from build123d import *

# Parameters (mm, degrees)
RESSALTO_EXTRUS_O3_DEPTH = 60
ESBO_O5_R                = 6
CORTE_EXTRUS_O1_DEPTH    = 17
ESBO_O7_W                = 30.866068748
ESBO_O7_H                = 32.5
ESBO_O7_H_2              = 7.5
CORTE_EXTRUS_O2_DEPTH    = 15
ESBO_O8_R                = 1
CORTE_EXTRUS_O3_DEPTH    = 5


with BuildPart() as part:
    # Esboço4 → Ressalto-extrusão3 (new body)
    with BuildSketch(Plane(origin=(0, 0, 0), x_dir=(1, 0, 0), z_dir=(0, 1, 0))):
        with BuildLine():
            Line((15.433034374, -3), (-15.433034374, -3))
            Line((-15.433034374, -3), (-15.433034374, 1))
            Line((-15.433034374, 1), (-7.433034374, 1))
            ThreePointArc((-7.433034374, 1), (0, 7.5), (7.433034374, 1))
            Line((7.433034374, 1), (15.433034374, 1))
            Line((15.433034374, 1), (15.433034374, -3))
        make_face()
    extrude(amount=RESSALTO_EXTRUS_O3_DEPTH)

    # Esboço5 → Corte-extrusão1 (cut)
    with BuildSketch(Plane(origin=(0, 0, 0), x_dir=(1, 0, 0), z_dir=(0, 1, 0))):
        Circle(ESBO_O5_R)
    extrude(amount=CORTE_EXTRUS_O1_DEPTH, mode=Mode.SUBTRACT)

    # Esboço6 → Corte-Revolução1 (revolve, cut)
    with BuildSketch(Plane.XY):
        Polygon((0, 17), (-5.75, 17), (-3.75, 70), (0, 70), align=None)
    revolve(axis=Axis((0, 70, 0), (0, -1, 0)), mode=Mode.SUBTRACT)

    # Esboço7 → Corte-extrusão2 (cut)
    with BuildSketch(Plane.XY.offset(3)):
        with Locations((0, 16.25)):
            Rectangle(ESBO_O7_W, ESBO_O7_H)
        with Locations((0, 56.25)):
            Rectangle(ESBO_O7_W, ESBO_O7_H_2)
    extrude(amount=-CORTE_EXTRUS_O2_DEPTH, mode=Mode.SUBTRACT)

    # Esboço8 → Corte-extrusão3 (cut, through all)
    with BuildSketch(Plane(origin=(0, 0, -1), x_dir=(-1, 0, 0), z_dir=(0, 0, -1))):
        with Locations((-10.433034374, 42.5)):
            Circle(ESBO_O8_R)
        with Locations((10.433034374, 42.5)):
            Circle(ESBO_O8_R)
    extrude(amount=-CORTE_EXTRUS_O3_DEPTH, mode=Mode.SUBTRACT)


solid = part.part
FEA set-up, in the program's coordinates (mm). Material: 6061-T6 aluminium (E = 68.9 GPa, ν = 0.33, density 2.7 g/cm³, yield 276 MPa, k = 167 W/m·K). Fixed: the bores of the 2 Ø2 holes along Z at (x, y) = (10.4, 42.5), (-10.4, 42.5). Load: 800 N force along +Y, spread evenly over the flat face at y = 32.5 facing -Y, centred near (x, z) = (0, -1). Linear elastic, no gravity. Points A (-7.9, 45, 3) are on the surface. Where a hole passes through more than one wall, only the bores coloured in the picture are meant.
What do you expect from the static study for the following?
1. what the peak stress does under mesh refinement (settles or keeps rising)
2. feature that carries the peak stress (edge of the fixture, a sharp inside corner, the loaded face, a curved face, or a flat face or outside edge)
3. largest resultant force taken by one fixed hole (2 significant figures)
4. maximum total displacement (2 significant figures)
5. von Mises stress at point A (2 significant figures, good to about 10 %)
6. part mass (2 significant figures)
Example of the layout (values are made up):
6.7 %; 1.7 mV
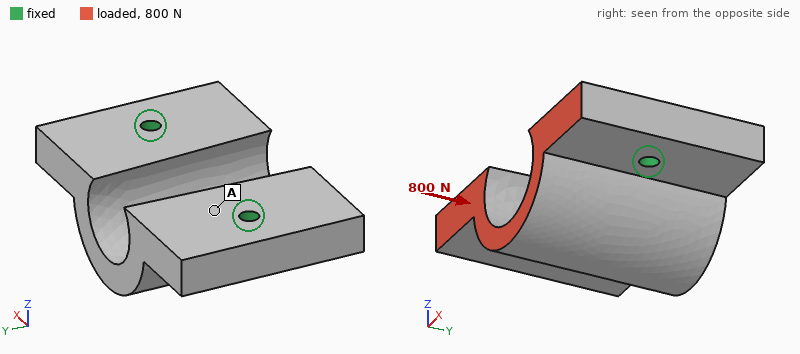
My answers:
keeps rising; edge of the fixture; 400 N; 13 µm; 6.3 MPa; 7.2 g
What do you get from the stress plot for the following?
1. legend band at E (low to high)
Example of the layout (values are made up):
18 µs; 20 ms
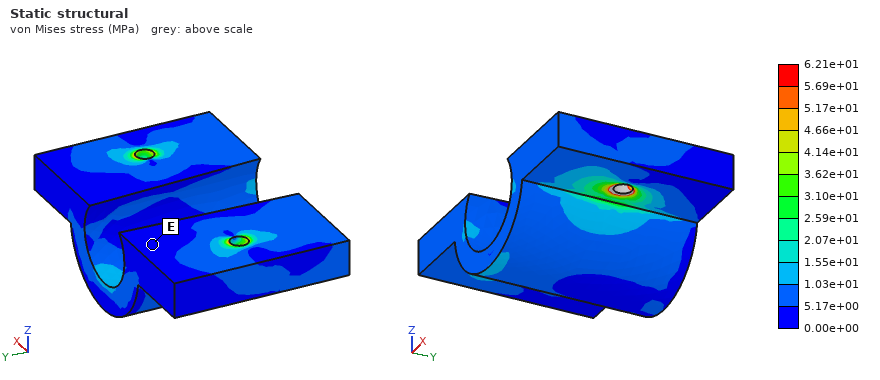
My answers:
0.00e+00 to 5.17e+00 MPa
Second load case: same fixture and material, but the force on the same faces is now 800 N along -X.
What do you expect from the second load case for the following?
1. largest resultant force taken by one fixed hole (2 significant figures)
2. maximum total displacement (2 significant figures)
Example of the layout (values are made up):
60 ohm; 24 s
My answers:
490 N; 19 µm
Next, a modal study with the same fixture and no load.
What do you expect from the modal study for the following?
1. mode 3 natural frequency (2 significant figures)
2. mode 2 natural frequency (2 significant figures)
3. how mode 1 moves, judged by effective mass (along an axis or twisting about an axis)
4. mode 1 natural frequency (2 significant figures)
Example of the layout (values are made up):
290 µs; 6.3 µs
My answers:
24 kHz; 22 kHz; along Y; 14 kHz
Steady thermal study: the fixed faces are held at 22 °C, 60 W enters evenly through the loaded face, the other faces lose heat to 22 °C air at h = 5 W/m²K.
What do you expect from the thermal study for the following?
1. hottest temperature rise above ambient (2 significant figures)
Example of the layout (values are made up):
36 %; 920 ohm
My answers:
40 K
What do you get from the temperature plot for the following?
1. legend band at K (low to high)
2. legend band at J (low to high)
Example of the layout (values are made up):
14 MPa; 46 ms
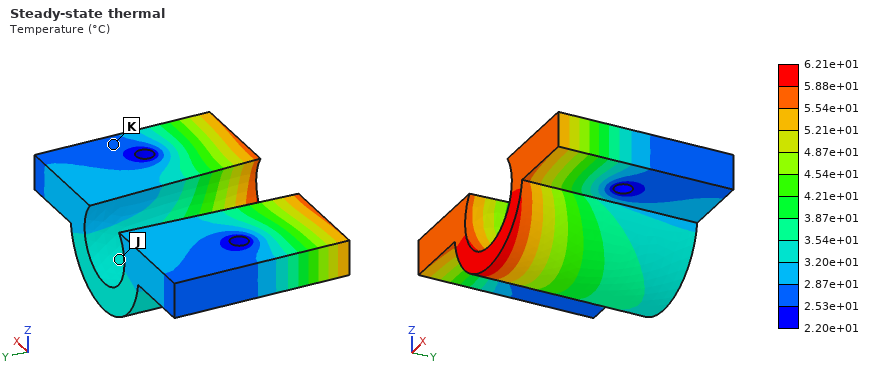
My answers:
2.53e+01 to 2.87e+01 °C; 3.20e+01 to 3.54e+01 °C
